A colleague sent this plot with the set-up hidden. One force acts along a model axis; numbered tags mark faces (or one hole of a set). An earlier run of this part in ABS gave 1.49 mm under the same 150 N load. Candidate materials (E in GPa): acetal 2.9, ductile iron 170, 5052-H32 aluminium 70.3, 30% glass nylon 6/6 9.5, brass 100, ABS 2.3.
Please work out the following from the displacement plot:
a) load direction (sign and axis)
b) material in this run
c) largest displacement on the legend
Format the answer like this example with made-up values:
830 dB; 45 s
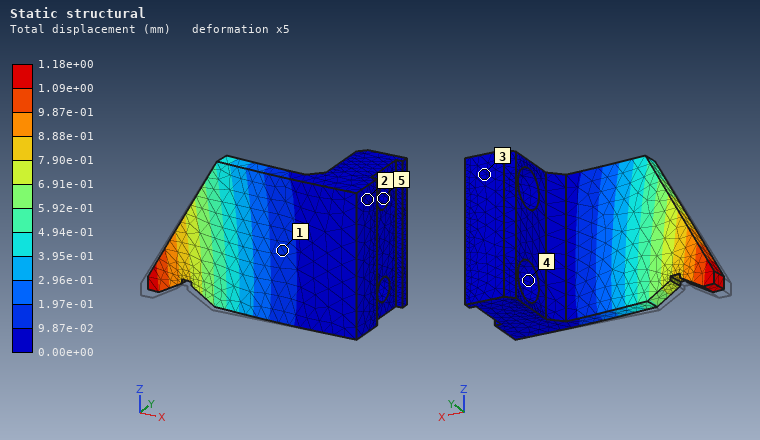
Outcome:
+Y; acetal; 1.18e+00 mm
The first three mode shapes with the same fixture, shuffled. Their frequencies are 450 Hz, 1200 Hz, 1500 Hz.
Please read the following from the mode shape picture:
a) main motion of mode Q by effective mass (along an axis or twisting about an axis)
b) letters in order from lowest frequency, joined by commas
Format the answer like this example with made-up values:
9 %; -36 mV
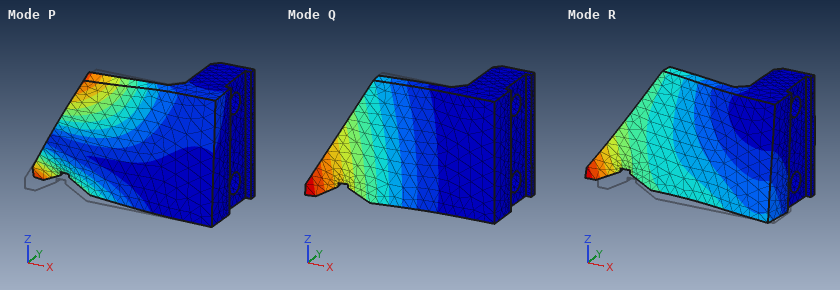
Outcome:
along Y; Q, P, R
